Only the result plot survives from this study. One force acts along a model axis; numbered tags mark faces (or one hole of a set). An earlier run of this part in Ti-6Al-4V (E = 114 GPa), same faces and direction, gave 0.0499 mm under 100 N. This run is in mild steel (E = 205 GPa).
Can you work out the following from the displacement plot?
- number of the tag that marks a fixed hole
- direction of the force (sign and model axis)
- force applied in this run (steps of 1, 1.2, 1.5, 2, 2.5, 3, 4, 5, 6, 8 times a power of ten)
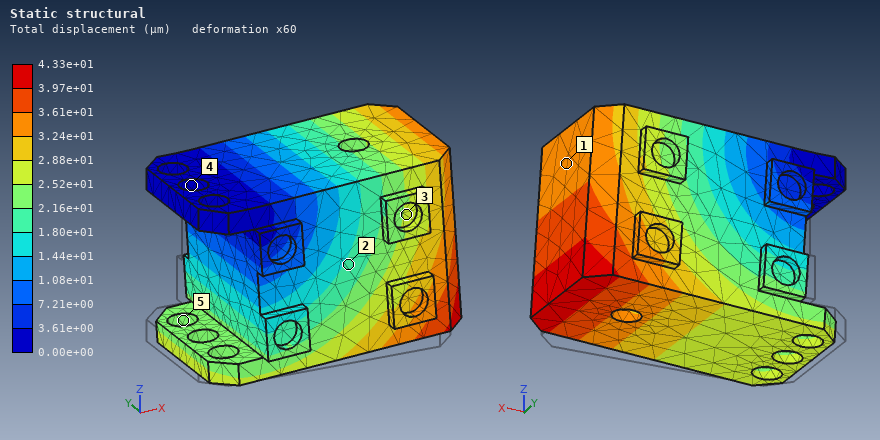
4
+X
150 N
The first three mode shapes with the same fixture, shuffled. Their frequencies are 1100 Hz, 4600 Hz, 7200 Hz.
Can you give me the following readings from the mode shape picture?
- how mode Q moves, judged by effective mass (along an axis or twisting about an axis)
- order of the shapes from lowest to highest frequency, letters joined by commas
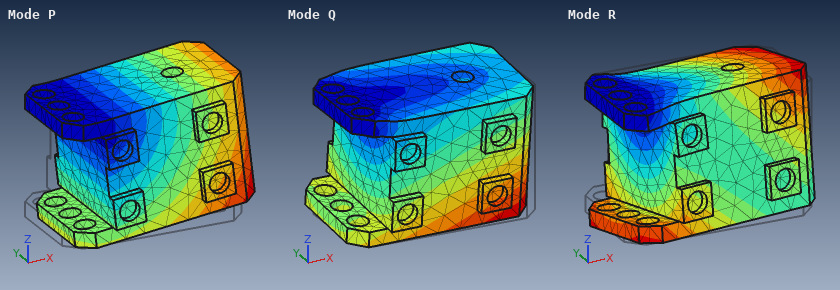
along Y
P, Q, R
